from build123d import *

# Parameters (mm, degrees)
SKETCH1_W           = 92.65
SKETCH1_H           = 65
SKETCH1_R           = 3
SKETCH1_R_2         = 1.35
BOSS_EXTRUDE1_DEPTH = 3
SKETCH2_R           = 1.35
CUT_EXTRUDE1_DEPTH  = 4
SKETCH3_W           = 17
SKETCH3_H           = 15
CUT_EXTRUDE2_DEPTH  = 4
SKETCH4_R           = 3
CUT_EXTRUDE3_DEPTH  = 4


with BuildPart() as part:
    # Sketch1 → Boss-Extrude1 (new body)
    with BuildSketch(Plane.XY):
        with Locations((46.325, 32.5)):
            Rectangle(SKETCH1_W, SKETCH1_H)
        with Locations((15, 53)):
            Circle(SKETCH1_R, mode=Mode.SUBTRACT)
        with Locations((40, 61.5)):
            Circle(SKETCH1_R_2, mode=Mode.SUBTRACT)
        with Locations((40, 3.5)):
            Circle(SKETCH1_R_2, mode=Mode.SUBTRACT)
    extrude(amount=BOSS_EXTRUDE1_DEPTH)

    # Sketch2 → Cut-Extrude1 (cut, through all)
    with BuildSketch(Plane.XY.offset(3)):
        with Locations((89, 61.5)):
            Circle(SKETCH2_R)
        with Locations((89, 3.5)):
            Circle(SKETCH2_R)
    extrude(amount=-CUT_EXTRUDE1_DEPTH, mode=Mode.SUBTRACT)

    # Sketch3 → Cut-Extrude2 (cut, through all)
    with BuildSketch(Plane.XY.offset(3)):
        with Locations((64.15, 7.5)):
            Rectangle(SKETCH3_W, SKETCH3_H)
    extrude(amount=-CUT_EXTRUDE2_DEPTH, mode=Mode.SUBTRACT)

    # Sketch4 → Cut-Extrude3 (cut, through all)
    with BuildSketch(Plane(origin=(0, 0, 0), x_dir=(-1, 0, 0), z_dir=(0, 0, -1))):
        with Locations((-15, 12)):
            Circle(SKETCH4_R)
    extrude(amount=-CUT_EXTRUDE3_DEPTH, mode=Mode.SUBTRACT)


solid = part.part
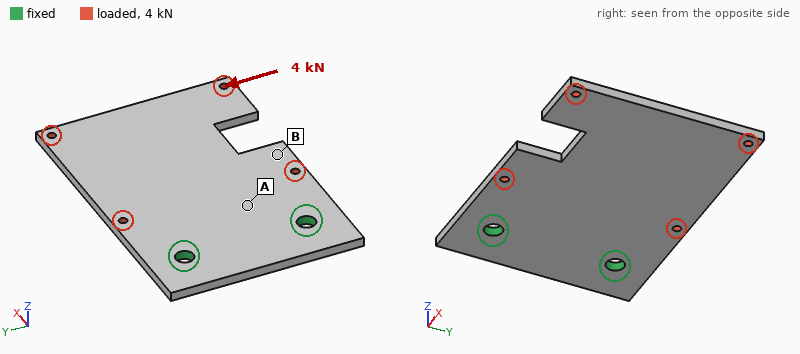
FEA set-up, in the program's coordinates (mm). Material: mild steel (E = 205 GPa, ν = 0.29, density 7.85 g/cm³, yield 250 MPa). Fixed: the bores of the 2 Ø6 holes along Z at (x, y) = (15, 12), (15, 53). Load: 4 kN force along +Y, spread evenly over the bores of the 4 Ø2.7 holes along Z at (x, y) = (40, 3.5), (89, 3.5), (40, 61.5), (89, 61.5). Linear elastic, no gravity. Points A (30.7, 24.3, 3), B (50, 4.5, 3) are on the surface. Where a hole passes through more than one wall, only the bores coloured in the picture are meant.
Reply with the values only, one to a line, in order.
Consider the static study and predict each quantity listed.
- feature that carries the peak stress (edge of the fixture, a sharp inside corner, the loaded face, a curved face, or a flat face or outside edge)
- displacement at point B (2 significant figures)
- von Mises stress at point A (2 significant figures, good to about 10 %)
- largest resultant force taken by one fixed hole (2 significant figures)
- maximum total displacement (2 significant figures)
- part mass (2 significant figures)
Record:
edge of the fixture
21 µm
59 MPa
5.0 kN
67 µm
130 g
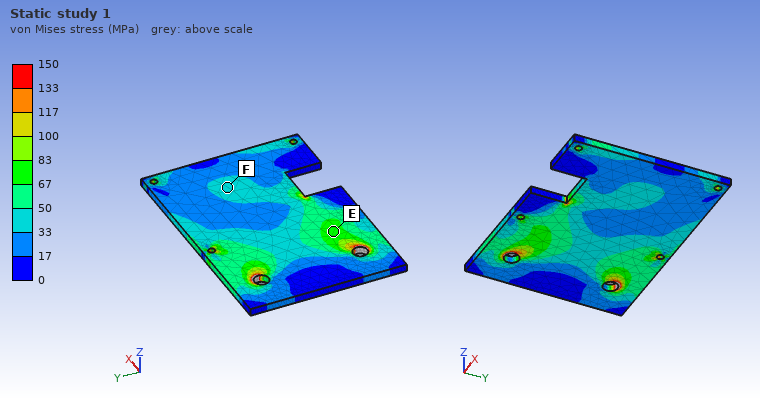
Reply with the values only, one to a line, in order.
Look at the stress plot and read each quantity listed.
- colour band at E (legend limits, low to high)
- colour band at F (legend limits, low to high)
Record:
67 to 83 MPa
33 to 50 MPa
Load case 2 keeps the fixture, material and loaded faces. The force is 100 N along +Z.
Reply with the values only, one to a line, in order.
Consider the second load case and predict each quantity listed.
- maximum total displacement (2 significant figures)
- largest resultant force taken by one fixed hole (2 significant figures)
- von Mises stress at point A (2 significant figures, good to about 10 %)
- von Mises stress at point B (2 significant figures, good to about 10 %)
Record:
0.30 mm
50 N
31 MPa
11 MPa
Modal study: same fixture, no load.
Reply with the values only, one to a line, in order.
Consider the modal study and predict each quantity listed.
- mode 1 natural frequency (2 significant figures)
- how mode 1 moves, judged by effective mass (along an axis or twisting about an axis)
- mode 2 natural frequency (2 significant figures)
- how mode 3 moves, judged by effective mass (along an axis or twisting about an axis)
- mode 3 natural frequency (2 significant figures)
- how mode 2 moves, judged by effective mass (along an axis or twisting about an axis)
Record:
420 Hz
along Z
1200 Hz
along Z
2500 Hz
twisting about X
